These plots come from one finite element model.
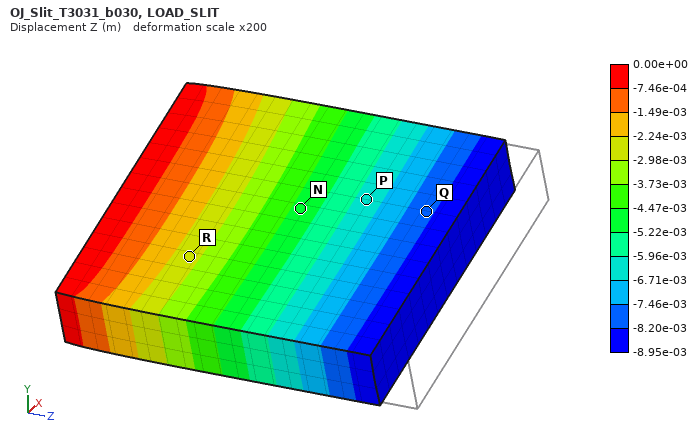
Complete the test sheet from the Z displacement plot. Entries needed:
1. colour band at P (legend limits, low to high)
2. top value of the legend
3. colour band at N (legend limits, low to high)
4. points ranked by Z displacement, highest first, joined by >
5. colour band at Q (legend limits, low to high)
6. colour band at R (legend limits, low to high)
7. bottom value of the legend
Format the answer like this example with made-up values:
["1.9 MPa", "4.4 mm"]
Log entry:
["-6.71e-03 to -5.96e-03 m", "0.00e+00 m", "-5.22e-03 to -4.47e-03 m", "R > N > P > Q", "-8.20e-03 to -7.46e-03 m", "-2.98e-03 to -2.24e-03 m", "-8.95e-03 m"]
